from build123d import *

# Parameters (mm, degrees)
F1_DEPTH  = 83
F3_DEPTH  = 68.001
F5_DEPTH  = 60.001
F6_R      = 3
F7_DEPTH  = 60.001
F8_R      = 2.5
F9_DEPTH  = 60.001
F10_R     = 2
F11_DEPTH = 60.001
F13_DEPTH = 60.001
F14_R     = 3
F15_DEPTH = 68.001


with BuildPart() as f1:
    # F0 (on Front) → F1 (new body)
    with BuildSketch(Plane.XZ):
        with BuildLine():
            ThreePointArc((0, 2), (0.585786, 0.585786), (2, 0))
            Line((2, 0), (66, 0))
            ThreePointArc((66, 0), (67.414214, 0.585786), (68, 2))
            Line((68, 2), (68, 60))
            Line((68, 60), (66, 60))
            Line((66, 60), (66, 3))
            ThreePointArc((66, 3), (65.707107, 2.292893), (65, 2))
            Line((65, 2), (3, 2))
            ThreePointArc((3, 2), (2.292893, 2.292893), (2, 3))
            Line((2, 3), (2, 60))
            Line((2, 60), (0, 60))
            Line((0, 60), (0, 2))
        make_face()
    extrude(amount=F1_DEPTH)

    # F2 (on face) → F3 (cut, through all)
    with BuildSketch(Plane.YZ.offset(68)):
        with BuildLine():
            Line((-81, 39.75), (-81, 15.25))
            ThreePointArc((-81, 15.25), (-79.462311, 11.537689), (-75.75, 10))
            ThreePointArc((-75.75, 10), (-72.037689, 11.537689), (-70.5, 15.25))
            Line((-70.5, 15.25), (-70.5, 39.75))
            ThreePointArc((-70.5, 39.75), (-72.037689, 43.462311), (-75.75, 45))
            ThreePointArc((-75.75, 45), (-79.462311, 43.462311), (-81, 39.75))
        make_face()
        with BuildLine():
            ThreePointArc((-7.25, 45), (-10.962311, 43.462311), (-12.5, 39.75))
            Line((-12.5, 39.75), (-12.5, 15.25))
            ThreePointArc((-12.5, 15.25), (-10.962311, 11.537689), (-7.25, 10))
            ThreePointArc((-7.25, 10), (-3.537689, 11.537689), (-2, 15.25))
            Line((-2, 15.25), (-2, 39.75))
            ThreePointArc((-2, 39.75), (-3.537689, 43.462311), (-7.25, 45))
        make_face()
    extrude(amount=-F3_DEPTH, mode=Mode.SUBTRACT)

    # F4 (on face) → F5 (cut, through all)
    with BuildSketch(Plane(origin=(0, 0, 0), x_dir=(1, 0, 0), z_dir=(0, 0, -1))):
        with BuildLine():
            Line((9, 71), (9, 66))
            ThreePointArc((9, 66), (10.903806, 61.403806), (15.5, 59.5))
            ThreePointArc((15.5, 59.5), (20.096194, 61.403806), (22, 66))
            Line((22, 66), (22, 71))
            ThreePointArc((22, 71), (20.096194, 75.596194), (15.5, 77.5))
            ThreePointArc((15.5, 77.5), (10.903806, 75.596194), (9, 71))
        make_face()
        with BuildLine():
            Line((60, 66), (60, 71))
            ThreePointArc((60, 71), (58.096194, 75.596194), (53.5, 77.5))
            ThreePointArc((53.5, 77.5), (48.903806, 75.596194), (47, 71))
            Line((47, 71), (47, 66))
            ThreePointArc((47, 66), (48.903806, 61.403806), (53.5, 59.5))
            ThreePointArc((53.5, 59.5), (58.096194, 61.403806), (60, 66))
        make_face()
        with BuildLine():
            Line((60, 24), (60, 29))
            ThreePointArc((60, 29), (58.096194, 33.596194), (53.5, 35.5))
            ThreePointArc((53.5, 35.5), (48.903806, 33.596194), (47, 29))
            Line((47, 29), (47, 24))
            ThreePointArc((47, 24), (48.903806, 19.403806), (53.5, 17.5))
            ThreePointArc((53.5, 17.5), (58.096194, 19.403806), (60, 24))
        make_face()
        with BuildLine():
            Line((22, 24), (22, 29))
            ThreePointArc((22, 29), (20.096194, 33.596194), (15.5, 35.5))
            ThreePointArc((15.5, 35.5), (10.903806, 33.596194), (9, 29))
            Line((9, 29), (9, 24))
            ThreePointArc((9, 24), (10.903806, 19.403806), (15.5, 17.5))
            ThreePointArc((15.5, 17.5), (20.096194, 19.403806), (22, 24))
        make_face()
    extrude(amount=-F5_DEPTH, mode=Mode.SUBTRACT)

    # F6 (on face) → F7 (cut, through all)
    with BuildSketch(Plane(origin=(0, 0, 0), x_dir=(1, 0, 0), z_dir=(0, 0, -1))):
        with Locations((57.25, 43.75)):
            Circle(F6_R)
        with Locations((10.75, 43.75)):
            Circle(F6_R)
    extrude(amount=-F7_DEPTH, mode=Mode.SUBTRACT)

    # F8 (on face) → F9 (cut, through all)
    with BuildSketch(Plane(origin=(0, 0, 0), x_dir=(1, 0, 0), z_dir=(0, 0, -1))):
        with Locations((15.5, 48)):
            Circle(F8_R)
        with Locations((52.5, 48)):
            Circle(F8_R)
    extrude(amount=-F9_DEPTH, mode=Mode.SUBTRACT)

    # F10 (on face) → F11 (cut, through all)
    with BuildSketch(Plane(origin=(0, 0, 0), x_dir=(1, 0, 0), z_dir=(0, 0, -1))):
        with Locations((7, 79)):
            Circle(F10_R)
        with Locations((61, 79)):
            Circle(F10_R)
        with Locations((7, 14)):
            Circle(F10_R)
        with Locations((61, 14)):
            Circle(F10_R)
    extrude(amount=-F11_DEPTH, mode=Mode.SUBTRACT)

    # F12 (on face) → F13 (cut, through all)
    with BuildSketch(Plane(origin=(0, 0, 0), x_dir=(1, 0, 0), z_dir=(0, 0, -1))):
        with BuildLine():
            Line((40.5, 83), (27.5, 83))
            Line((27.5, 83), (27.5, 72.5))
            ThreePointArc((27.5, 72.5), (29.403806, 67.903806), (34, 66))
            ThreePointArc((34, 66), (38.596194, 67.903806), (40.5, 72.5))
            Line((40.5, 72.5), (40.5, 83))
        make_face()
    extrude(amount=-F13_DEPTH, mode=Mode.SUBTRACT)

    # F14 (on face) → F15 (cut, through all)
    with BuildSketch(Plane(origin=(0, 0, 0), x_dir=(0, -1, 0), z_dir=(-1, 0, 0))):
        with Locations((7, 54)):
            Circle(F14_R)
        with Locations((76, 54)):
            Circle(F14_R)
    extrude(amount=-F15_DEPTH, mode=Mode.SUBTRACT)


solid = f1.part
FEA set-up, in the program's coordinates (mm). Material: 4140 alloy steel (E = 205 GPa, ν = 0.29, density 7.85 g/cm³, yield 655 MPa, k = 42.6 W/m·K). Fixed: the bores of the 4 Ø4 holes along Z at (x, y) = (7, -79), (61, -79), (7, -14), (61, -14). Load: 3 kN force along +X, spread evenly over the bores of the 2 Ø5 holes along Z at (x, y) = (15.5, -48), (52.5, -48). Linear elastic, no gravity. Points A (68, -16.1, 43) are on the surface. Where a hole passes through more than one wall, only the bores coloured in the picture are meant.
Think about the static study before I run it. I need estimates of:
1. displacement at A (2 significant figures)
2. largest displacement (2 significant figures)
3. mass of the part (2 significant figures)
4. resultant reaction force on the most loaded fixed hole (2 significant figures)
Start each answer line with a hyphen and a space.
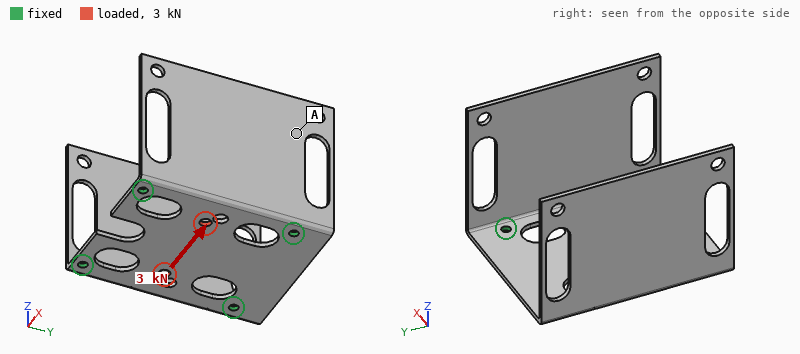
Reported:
- 5.1 µm
- 18 µm
- 200 g
- 930 N
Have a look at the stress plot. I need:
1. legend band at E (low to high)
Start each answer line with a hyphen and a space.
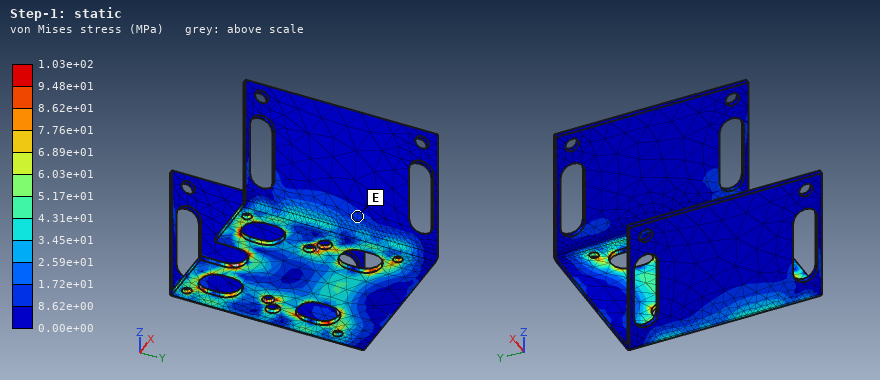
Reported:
- 8.62e+00 to 1.72e+01 MPa
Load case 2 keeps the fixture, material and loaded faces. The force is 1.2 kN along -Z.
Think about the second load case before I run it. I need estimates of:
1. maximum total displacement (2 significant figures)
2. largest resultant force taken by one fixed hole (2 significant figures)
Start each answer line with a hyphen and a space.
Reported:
- 0.37 mm
- 360 N
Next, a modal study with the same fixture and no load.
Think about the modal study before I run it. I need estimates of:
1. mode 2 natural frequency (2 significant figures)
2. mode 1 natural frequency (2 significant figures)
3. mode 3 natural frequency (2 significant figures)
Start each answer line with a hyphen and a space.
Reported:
- 380 Hz
- 370 Hz
- 880 Hz
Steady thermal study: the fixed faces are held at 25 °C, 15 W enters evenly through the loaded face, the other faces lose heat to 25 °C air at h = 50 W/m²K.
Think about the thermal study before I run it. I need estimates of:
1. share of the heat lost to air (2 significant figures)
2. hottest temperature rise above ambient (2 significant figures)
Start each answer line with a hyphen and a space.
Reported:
- 71 %
- 54 K
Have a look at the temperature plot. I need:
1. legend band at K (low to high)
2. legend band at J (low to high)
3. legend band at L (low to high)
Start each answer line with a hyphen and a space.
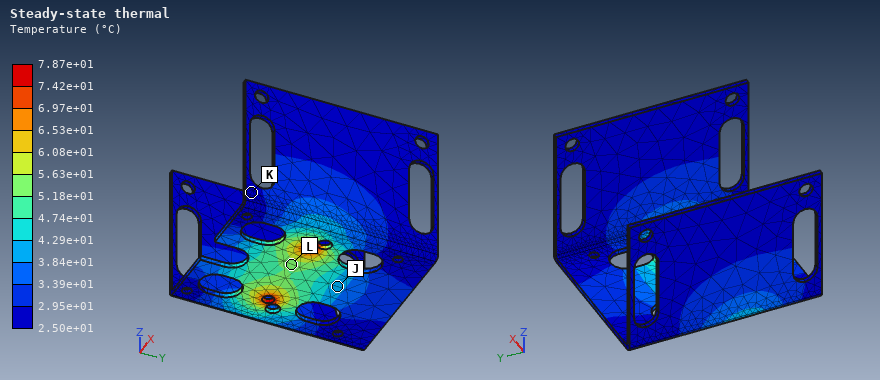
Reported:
- 2.50e+01 to 2.95e+01 °C
- 3.84e+01 to 4.29e+01 °C
- 5.18e+01 to 5.63e+01 °C
